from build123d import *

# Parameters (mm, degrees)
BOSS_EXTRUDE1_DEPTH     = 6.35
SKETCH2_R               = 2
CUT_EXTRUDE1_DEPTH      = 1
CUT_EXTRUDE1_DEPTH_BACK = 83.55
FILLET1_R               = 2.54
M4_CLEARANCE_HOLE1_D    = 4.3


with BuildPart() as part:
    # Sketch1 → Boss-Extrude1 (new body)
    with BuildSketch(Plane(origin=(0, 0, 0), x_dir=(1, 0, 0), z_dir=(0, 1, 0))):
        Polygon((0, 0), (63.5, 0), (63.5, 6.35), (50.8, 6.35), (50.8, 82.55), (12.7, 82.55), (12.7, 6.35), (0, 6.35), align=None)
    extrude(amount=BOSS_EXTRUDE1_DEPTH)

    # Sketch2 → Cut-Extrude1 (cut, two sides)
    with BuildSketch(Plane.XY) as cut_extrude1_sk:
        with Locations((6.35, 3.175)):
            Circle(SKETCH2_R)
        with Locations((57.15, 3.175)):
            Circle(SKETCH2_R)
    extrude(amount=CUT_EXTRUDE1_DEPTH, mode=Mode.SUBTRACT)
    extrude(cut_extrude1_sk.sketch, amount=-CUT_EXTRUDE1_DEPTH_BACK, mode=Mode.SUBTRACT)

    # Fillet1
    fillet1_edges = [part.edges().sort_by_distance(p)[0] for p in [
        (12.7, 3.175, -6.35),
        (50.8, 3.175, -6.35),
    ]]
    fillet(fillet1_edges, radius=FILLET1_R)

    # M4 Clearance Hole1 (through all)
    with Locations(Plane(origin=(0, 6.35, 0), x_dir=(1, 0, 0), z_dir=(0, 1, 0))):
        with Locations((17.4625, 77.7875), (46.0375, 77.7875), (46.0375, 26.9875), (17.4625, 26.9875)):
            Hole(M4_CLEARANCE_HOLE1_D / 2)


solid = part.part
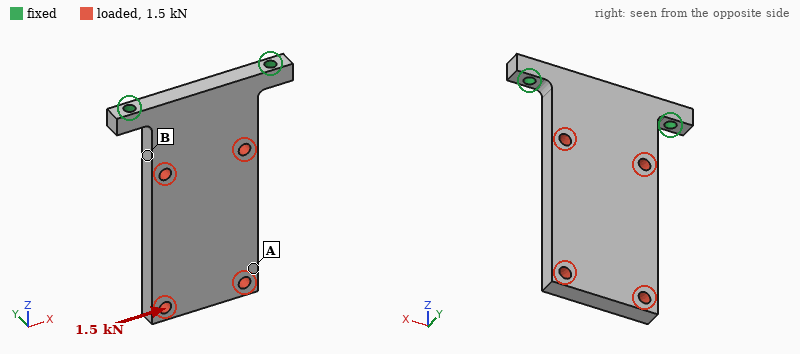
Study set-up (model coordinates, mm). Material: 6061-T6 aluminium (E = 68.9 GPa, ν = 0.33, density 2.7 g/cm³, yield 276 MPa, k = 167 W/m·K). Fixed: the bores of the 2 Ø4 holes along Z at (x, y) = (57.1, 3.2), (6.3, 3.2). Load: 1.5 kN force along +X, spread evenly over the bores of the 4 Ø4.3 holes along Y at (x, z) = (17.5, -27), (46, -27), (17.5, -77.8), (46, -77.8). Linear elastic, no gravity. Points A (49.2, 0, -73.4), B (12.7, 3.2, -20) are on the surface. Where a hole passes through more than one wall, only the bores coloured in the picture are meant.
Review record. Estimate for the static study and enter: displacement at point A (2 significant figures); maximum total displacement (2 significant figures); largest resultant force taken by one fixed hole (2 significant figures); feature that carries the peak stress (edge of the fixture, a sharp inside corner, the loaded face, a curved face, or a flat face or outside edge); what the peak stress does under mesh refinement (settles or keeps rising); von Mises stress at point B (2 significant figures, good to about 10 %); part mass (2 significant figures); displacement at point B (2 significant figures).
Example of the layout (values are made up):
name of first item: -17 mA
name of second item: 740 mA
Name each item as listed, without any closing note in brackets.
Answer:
displacement at point A: 0.13 mm
maximum total displacement: 0.15 mm
largest resultant force taken by one fixed hole: 1.9 kN
feature that carries the peak stress: edge of the fixture
what the peak stress does under mesh refinement: keeps rising
von Mises stress at point B: 38 MPa
part mass: 55 g
displacement at point B: 0.032 mm
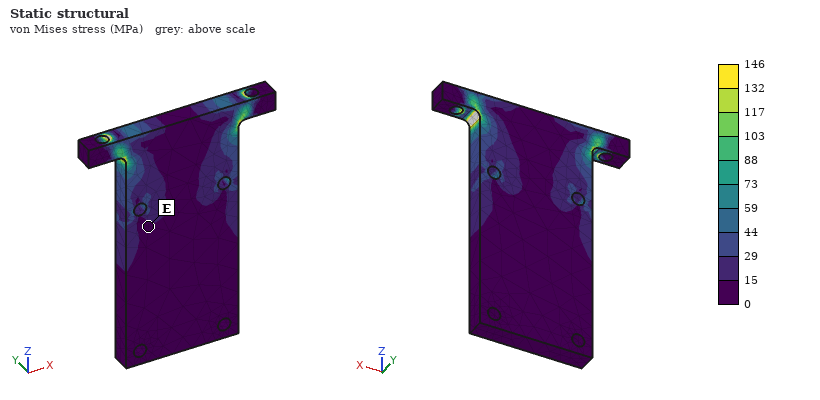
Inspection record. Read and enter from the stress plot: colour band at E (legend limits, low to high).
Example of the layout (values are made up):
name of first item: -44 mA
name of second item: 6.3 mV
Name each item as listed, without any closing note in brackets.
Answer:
colour band at E: 0 to 15 MPa
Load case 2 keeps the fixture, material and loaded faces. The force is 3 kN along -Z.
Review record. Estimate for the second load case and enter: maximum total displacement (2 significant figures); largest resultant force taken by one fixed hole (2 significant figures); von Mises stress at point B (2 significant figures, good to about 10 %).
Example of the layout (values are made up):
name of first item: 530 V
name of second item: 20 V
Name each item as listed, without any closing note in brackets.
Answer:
maximum total displacement: 29 µm
largest resultant force taken by one fixed hole: 1.7 kN
von Mises stress at point B: 20 MPa
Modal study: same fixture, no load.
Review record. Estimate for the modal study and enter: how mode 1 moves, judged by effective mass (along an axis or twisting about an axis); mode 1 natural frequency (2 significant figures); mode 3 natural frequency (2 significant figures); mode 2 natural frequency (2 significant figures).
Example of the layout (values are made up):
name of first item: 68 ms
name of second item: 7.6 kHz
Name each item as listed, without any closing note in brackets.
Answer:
how mode 1 moves, judged by effective mass: along Y
mode 1 natural frequency: 510 Hz
mode 3 natural frequency: 3200 Hz
mode 2 natural frequency: 3200 Hz
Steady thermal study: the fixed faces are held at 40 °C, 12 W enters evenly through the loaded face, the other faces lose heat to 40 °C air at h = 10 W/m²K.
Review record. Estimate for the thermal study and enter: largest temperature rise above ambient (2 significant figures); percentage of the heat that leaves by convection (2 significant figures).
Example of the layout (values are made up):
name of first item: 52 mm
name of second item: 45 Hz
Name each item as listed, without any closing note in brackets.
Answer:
largest temperature rise above ambient: 21 K
percentage of the heat that leaves by convection: 9.2 %
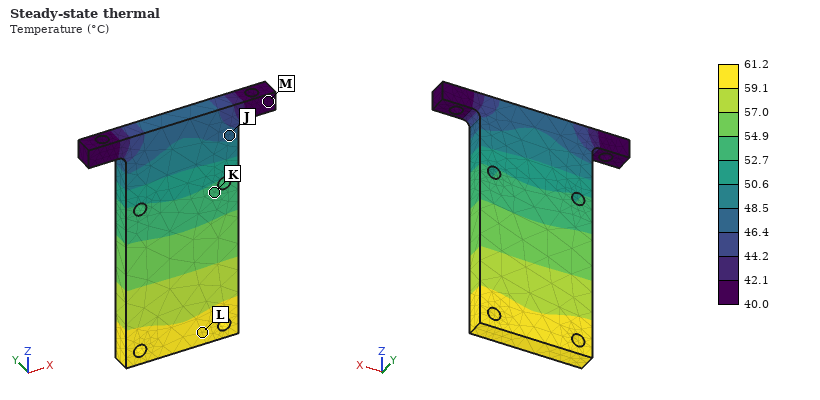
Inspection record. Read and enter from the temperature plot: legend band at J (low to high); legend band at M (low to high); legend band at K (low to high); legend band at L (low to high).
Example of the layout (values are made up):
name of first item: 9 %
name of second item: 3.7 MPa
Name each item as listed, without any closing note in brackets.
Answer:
legend band at J: 46.4 to 48.5 °C
legend band at M: 40.0 to 42.1 °C
legend band at K: 52.7 to 54.9 °C
legend band at L: 59.1 to 61.2 °C
